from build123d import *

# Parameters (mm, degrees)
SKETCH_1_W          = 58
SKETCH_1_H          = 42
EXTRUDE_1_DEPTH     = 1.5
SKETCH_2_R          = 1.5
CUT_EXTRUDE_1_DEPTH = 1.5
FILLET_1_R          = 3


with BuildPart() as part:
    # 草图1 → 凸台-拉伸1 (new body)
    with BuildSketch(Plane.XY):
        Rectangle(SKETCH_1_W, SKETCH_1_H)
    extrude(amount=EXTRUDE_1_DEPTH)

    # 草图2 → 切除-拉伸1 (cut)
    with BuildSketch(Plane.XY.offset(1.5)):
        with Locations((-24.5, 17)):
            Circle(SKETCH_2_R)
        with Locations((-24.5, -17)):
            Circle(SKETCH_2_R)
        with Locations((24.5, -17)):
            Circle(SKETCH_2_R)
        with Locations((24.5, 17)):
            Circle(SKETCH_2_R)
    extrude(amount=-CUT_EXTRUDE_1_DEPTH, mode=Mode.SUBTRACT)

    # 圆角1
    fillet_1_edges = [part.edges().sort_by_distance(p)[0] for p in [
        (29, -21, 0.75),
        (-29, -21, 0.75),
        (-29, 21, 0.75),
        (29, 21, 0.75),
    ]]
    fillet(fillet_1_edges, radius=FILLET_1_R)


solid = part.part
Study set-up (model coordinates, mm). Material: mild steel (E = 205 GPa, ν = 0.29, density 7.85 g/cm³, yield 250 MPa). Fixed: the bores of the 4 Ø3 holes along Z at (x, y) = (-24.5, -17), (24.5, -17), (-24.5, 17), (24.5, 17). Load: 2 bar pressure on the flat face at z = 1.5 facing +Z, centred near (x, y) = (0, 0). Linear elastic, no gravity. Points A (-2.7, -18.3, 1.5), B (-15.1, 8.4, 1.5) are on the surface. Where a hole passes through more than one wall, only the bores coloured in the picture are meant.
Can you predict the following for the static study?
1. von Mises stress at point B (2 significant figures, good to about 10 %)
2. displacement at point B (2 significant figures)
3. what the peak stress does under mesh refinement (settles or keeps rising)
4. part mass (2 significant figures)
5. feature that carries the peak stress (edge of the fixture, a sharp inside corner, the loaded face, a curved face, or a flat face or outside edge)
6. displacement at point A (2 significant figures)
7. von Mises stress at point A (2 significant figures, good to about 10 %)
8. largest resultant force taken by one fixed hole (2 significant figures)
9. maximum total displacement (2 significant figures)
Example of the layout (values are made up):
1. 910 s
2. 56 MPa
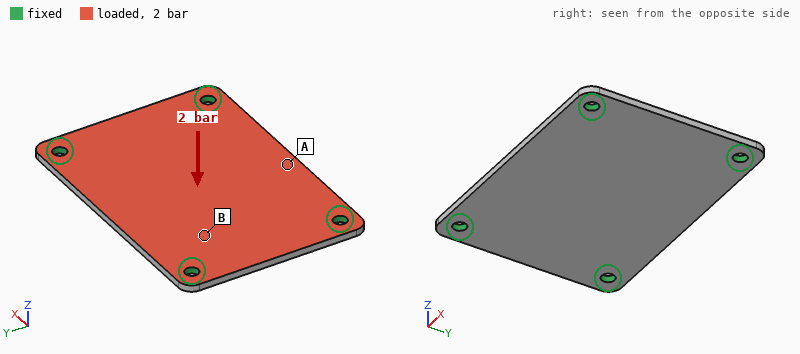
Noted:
1. 20 MPa
2. 37 µm
3. keeps rising
4. 28 g
5. edge of the fixture
6. 60 µm
7. 61 MPa
8. 120 N
9. 73 µm
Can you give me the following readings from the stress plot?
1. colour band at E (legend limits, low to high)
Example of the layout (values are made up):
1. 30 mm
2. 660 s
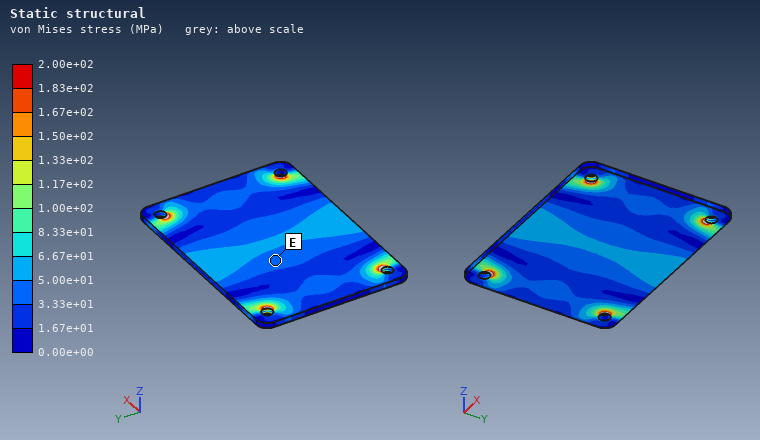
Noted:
1. 3.33e+01 to 5.00e+01 MPa
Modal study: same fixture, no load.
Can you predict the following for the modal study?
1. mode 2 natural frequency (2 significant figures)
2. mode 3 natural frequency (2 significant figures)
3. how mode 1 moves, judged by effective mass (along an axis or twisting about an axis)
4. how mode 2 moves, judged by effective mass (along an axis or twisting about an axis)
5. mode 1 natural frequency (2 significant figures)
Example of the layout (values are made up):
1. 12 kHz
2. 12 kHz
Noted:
1. 4300 Hz
2. 6500 Hz
3. along Z
4. twisting about X
5. 2900 Hz
